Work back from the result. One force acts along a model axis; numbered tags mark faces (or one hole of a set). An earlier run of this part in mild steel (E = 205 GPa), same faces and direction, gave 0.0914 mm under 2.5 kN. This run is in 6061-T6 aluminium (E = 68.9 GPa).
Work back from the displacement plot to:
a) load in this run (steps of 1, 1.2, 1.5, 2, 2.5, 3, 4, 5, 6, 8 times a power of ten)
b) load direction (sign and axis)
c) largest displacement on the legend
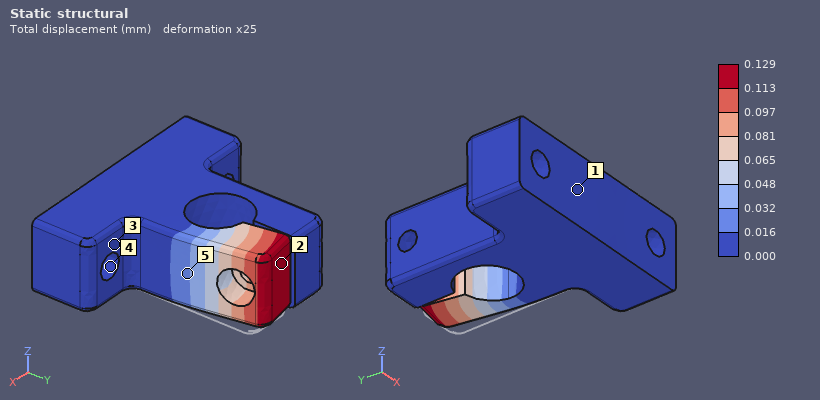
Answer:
1.2 kN
-X
0.129 mm
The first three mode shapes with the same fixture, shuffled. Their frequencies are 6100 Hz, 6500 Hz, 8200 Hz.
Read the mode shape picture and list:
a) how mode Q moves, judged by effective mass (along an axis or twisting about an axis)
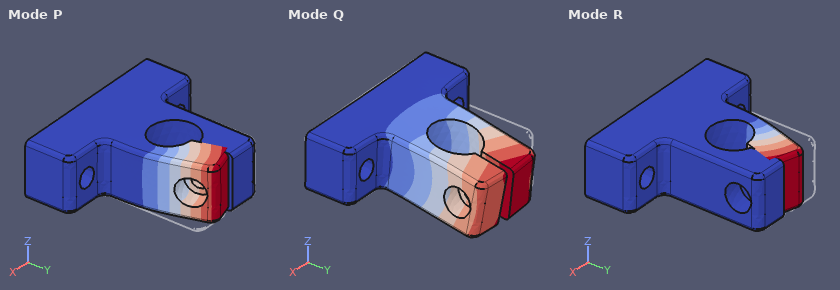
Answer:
along Z
